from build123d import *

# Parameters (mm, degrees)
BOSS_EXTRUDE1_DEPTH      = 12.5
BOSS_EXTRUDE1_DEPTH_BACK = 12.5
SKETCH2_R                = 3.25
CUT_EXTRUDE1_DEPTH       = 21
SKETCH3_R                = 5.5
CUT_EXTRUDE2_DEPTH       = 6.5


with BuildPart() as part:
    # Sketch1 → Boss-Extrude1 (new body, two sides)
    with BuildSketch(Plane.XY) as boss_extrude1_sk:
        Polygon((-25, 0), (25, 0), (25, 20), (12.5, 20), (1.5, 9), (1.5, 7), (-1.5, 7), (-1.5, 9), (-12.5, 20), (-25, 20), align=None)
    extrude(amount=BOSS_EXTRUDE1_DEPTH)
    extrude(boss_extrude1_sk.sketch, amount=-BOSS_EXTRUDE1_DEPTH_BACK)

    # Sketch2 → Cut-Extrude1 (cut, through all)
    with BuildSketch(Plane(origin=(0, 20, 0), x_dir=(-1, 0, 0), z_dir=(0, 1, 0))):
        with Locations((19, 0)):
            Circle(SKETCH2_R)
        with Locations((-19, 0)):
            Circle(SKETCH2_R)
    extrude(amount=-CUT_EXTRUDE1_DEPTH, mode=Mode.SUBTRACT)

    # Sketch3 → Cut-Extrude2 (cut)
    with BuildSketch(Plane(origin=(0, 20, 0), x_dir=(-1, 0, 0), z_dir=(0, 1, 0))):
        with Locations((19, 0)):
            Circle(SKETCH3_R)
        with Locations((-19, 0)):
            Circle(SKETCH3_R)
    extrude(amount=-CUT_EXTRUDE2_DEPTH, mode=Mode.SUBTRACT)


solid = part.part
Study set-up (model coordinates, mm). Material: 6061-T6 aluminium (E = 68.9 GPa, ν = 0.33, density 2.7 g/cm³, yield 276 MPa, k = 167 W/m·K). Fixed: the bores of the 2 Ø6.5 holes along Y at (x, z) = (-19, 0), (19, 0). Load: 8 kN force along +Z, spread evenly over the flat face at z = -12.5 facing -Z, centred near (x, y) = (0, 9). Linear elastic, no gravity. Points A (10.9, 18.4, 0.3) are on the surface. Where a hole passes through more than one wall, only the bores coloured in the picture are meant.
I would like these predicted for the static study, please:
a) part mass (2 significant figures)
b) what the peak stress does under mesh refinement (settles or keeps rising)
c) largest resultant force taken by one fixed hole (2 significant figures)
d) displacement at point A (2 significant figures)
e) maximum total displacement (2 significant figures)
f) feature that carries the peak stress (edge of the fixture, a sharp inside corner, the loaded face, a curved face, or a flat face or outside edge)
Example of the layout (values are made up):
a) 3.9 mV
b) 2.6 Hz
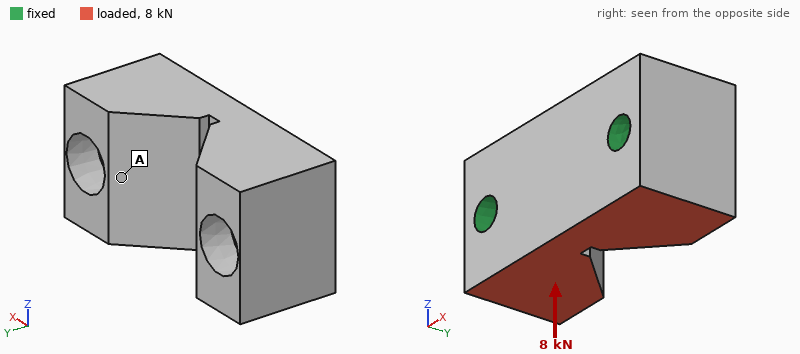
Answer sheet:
a) 51 g
b) keeps rising
c) 4.0 kN
d) 4.3 µm
e) 7.4 µm
f) edge of the fixture
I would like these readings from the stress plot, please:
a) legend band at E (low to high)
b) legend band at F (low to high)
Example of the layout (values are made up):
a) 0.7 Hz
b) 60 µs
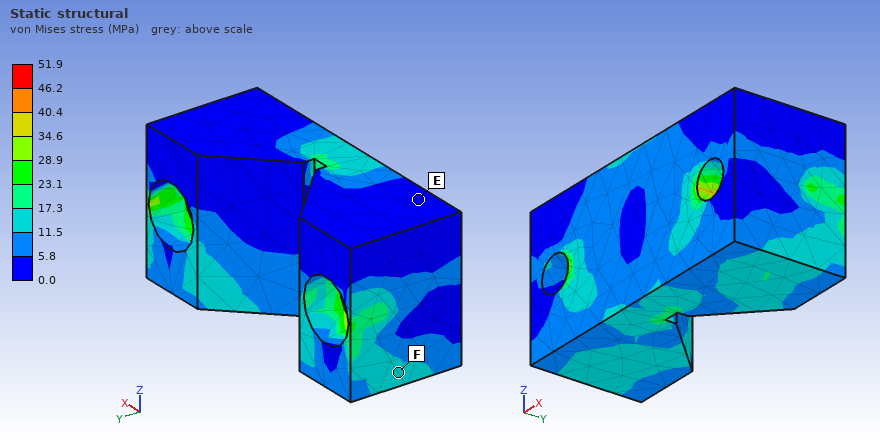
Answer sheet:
a) 0.0 to 5.8 MPa
b) 11.5 to 17.3 MPa
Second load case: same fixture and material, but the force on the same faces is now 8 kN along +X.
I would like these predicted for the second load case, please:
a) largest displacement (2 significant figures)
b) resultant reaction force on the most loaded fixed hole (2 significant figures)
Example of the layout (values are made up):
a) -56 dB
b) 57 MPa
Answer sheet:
a) 13 µm
b) 4.5 kN
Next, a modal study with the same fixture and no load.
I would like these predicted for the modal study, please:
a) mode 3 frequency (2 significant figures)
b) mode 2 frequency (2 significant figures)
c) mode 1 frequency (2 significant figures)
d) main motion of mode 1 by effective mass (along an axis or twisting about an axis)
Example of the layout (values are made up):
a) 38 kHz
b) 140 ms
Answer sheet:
a) 28 kHz
b) 27 kHz
c) 25 kHz
d) along Y
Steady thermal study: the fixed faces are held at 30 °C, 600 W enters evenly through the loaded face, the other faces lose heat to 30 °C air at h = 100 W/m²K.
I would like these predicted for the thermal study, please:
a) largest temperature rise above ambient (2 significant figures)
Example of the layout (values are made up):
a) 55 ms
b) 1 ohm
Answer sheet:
a) 73 K
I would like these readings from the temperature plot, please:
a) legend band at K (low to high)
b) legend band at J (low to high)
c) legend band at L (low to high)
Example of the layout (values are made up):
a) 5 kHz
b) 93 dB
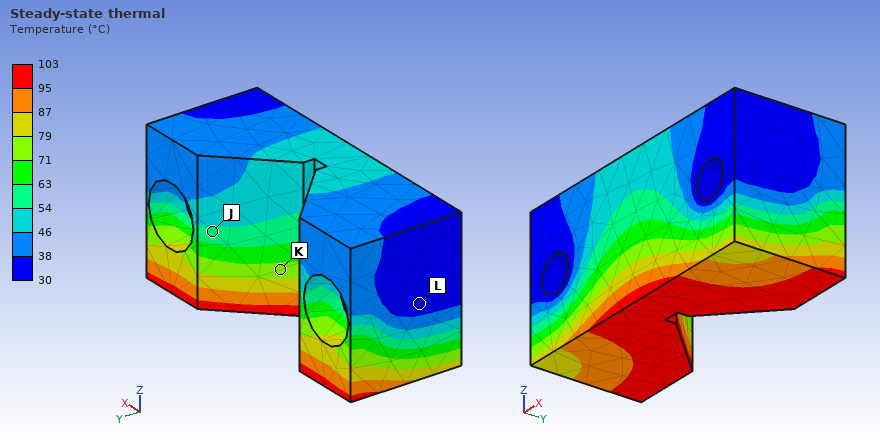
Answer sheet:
a) 71 to 79 °C
b) 54 to 63 °C
c) 30 to 38 °C
